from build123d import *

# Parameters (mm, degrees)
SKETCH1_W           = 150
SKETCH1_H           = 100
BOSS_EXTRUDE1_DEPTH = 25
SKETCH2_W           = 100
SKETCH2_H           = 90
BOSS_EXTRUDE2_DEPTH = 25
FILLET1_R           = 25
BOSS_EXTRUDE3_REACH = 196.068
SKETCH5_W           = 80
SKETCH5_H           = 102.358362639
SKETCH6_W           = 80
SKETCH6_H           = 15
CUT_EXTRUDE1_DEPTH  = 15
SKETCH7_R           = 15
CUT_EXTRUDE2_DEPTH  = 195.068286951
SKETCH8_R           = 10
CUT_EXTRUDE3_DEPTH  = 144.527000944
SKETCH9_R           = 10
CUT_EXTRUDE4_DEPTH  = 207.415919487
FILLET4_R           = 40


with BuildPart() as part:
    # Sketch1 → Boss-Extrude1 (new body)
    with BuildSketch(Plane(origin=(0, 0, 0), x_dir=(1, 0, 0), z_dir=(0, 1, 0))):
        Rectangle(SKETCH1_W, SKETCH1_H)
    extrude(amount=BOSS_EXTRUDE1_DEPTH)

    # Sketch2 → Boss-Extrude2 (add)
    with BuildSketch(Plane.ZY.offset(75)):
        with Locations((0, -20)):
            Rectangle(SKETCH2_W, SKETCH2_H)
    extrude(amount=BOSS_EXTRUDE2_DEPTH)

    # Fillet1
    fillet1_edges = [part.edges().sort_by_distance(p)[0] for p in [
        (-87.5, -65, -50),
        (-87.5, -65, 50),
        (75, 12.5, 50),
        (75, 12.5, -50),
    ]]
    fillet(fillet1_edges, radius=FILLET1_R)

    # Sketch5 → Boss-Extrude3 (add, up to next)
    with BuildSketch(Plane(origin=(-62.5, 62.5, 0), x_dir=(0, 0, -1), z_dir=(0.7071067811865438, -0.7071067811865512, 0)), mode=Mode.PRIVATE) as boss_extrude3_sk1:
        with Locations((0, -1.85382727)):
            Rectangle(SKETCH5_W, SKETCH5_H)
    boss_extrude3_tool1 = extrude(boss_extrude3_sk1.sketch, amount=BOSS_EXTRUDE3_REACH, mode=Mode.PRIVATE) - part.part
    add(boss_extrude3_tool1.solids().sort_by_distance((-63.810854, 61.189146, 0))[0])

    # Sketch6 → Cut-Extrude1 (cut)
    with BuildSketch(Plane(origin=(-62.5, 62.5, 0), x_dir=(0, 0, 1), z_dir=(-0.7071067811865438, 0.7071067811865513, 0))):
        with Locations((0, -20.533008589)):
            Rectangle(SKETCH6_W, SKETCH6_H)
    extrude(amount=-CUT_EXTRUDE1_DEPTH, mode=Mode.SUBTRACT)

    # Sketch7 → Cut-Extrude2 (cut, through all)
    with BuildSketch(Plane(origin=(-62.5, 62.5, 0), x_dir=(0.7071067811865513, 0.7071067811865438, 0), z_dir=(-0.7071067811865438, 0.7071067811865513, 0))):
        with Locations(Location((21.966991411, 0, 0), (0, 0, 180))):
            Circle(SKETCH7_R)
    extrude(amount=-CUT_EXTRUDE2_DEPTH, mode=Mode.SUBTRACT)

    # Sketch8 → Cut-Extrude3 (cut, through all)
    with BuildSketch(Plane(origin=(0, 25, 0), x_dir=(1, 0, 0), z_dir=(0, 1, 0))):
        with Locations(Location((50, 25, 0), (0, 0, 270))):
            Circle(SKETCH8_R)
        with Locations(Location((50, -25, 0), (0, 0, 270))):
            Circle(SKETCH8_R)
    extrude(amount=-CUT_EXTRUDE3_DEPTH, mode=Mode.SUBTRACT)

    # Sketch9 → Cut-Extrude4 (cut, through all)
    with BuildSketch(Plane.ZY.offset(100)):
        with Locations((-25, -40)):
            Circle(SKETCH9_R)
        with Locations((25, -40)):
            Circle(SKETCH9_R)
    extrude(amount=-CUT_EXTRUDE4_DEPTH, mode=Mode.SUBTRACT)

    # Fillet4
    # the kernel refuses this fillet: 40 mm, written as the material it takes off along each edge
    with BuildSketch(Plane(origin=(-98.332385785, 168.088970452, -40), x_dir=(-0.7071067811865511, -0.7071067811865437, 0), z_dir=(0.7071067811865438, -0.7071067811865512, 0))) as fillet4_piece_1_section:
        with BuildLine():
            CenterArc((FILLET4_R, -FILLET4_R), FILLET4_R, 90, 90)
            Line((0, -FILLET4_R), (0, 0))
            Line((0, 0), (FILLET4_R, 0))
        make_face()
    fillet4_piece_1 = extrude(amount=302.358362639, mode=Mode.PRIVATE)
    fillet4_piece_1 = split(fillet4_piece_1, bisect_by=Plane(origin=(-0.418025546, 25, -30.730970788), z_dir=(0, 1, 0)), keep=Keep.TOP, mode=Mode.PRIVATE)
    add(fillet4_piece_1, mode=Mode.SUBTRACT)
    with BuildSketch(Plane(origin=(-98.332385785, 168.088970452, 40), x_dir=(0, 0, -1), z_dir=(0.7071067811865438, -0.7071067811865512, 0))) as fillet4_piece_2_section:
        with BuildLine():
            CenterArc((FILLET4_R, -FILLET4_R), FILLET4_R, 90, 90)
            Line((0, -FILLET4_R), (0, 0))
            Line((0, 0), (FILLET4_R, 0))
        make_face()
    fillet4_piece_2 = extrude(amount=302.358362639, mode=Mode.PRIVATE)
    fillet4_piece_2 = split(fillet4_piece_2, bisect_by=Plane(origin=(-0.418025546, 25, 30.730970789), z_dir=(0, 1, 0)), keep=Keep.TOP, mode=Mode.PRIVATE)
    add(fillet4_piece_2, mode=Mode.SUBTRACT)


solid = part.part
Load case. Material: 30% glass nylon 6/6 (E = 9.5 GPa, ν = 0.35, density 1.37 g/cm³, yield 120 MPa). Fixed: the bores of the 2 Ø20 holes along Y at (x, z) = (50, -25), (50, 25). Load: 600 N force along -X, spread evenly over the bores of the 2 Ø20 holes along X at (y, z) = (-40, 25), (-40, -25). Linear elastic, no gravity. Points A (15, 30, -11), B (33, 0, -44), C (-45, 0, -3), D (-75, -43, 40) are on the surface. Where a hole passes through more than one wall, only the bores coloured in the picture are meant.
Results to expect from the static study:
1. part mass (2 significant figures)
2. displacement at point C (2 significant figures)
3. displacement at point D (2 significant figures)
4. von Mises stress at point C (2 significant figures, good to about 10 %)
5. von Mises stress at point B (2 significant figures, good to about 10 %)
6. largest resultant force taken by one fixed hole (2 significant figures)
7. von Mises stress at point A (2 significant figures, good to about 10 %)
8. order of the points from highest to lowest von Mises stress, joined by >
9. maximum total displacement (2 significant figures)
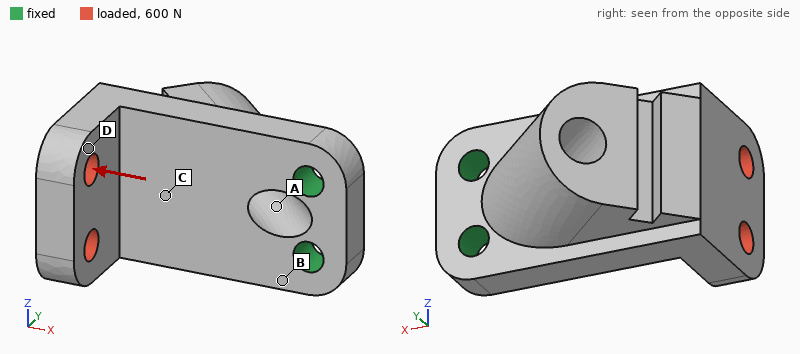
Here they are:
1.1 kg
0.067 mm
0.14 mm
1.2 MPa
2.4 MPa
320 N
0.79 MPa
B > C > A > D
0.20 mm
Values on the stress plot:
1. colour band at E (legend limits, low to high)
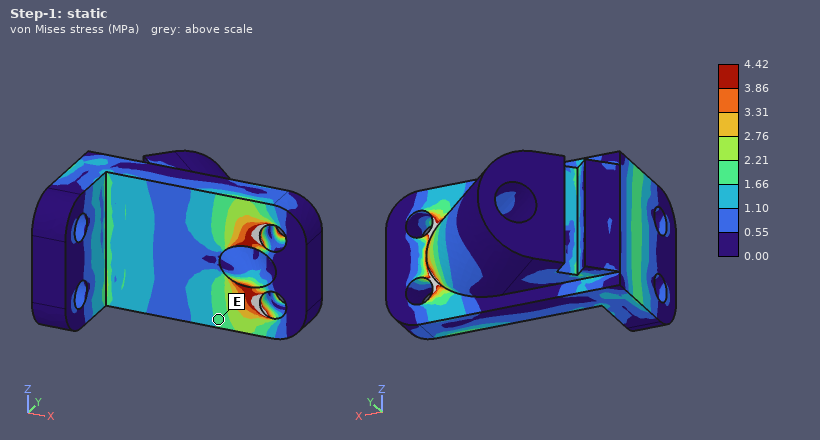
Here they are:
1.66 to 2.21 MPa
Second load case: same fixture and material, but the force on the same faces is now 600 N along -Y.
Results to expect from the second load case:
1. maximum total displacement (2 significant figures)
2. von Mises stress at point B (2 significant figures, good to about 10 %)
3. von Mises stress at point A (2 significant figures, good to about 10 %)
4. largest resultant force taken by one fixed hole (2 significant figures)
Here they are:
0.30 mm
5.1 MPa
2.2 MPa
400 N
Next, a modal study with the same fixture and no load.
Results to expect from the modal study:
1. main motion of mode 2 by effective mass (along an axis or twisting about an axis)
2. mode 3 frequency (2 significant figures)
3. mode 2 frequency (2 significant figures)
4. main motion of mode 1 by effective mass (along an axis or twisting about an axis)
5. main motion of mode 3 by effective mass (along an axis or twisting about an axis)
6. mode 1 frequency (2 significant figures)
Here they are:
along Z
1200 Hz
750 Hz
along Y
along Z
340 Hz
